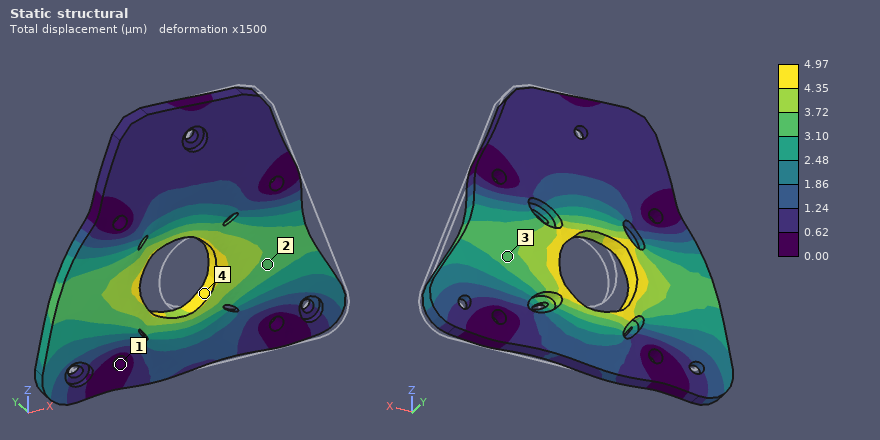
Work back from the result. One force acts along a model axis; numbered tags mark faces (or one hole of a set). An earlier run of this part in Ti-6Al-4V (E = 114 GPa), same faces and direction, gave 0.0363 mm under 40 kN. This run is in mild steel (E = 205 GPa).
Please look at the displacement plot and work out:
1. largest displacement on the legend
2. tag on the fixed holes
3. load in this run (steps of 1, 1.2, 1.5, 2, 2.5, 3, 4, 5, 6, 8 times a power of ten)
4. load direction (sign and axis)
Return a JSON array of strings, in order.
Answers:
["4.97 µm", "1", "10 kN", "-X"]
